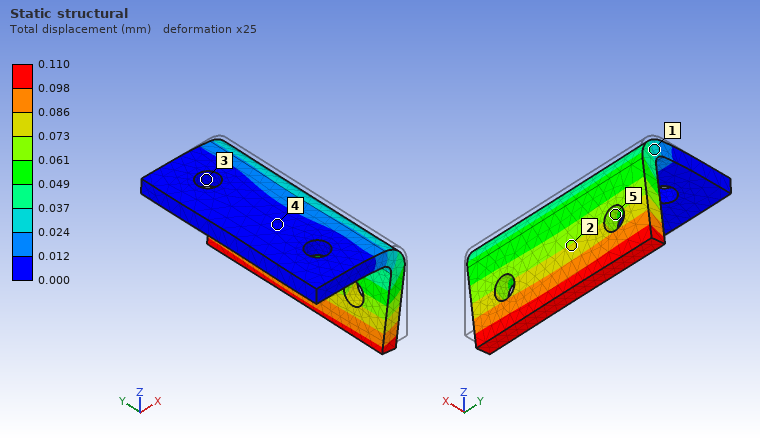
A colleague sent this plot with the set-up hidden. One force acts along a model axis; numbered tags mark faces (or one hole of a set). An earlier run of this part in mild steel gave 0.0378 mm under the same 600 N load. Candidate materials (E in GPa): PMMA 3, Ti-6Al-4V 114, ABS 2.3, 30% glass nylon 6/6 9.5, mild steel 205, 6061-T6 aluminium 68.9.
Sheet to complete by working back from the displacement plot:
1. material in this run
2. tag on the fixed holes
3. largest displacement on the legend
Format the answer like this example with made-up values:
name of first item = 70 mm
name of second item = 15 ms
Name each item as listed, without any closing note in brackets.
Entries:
material in this run = 6061-T6 aluminium
tag on the fixed holes = 3
largest displacement on the legend = 0.110 mm
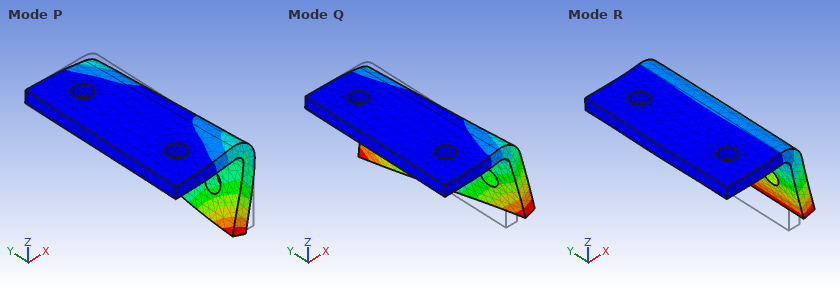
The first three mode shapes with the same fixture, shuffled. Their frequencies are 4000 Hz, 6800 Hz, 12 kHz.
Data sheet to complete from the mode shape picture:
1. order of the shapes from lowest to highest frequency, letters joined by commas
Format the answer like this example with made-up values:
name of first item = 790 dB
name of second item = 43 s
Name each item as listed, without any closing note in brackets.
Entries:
order of the shapes from lowest to highest frequency, letters joined by commas = R, Q, P
